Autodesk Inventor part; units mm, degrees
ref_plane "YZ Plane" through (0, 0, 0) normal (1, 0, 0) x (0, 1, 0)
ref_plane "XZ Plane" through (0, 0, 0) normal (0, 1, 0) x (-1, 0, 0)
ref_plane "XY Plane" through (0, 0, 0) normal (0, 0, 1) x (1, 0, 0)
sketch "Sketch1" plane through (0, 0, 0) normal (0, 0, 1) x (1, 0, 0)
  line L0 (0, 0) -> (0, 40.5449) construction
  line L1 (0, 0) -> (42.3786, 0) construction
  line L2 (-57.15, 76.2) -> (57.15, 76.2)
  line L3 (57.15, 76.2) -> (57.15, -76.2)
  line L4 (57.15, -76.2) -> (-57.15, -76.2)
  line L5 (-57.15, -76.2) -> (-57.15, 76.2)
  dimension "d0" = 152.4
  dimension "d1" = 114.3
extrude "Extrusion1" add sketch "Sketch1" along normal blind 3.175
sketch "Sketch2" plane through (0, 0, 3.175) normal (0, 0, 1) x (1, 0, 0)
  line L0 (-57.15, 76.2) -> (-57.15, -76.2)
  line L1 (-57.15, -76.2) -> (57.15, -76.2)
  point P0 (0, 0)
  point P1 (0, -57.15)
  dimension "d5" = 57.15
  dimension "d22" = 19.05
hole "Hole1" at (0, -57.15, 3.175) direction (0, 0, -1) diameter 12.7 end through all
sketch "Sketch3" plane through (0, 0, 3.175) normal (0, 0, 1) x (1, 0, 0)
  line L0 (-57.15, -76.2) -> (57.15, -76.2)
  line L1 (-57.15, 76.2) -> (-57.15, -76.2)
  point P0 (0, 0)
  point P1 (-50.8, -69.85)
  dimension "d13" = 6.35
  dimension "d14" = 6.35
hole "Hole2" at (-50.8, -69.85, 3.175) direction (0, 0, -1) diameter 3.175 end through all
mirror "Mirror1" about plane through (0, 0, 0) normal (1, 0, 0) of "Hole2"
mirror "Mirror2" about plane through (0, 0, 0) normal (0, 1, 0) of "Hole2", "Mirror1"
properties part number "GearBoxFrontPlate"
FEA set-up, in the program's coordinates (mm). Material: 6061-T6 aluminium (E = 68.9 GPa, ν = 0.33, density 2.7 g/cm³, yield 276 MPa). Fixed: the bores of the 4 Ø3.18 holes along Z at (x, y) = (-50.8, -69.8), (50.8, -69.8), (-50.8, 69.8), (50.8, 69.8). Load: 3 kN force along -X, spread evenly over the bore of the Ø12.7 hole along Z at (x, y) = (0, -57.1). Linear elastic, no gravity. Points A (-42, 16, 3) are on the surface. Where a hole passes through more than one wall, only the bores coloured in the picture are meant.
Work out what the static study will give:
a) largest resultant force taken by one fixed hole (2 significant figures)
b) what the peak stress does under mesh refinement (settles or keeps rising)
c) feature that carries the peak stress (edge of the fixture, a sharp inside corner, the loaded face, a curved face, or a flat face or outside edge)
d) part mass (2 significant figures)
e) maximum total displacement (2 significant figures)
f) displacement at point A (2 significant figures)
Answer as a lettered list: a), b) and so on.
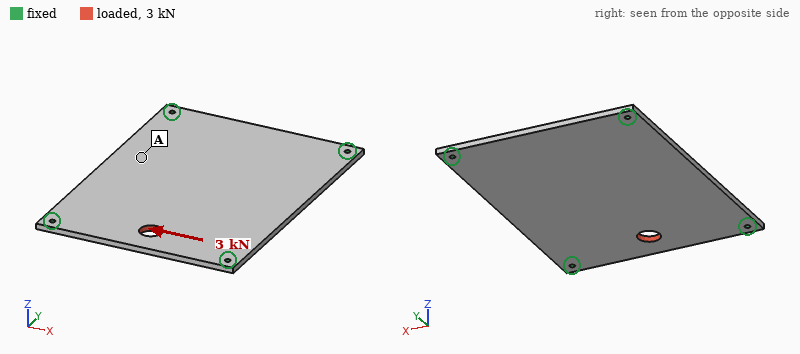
a) 1.3 kN
b) keeps rising
c) edge of the fixture
d) 150 g
e) 16 µm
f) 5.8 µm
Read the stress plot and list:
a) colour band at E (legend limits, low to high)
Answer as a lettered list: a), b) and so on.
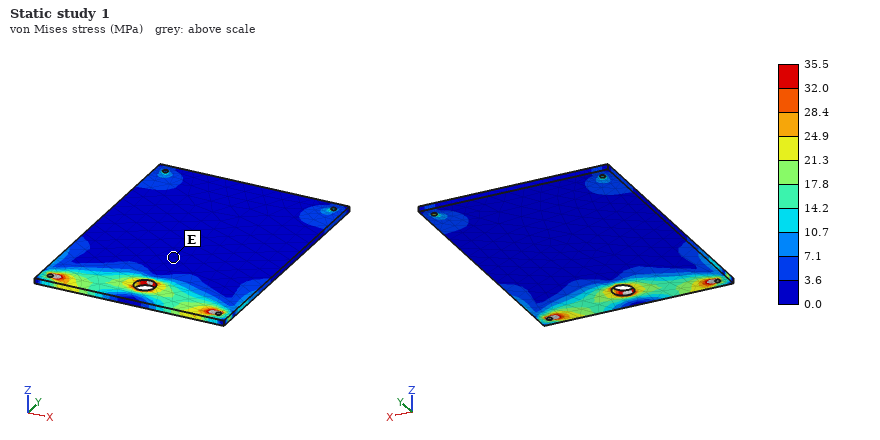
a) 0.0 to 3.6 MPa
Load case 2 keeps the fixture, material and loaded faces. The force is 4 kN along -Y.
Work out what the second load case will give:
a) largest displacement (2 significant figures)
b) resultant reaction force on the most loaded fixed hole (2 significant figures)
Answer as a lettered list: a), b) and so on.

a) 34 µm
b) 1.3 kN
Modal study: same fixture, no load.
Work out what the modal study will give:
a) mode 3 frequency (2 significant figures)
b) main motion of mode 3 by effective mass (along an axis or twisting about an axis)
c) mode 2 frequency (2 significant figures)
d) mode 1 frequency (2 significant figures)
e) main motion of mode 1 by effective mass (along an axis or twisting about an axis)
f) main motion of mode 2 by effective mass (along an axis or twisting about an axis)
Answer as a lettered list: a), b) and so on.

a) 1400 Hz
b) twisting about X
c) 1000 Hz
d) 610 Hz
e) along Z
f) twisting about Y
